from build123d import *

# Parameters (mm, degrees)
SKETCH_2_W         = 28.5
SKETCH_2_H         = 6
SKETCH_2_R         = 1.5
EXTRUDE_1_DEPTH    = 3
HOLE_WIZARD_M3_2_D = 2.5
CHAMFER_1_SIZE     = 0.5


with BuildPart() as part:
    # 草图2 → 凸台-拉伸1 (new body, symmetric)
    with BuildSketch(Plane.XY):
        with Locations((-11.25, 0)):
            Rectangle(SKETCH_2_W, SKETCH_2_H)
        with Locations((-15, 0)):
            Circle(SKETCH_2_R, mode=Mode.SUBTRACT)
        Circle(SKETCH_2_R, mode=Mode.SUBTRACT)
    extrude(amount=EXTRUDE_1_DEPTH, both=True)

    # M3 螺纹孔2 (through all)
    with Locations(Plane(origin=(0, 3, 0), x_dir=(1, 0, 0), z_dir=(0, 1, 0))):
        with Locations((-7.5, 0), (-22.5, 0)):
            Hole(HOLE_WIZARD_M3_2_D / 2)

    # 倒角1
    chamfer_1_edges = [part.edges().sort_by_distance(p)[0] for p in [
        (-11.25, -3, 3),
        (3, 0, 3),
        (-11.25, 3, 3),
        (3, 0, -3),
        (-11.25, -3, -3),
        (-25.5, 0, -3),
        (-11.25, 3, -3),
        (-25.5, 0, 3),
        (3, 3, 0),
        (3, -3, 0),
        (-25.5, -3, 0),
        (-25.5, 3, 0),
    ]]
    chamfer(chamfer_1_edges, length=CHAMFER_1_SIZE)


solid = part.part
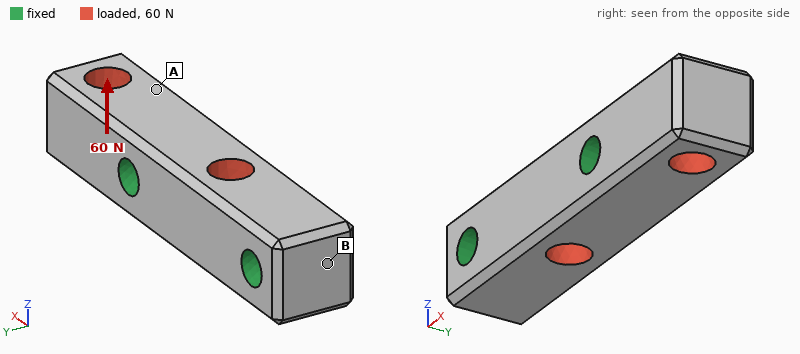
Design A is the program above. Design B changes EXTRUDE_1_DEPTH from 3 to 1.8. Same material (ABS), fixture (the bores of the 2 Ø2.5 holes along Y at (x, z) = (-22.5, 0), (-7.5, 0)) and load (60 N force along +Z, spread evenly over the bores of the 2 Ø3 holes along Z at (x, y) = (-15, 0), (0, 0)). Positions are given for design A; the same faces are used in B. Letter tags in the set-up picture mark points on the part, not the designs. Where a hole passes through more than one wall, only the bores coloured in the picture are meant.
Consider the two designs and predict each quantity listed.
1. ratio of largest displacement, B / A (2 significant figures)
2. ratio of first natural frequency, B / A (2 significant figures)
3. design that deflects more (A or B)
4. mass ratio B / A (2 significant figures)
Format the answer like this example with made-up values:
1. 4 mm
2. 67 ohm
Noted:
1. 2.9
2. 0.82
3. B
4. 0.56
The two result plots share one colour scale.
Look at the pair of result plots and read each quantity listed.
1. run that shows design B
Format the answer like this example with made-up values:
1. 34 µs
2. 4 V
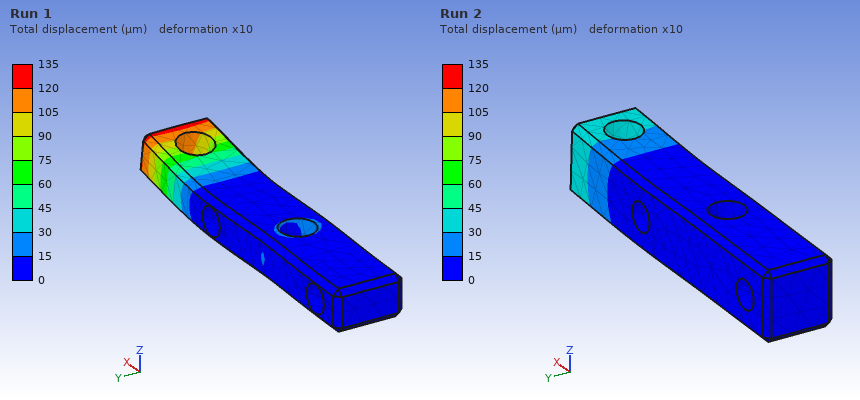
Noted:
1. Run 1
